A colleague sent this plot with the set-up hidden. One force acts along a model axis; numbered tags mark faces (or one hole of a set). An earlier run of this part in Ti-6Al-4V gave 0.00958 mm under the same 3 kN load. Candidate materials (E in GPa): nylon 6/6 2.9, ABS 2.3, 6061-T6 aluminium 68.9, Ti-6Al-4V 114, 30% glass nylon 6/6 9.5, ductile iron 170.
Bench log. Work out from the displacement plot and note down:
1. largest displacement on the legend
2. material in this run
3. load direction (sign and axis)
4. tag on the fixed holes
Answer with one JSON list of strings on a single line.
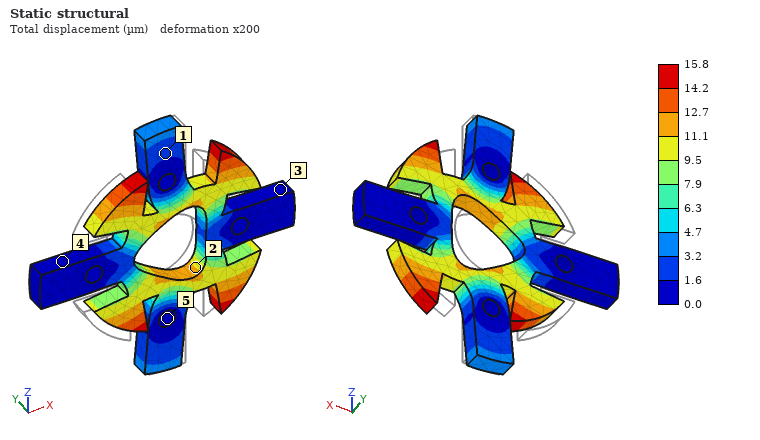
["15.8 µm", "6061-T6 aluminium", "+X", "5"]
